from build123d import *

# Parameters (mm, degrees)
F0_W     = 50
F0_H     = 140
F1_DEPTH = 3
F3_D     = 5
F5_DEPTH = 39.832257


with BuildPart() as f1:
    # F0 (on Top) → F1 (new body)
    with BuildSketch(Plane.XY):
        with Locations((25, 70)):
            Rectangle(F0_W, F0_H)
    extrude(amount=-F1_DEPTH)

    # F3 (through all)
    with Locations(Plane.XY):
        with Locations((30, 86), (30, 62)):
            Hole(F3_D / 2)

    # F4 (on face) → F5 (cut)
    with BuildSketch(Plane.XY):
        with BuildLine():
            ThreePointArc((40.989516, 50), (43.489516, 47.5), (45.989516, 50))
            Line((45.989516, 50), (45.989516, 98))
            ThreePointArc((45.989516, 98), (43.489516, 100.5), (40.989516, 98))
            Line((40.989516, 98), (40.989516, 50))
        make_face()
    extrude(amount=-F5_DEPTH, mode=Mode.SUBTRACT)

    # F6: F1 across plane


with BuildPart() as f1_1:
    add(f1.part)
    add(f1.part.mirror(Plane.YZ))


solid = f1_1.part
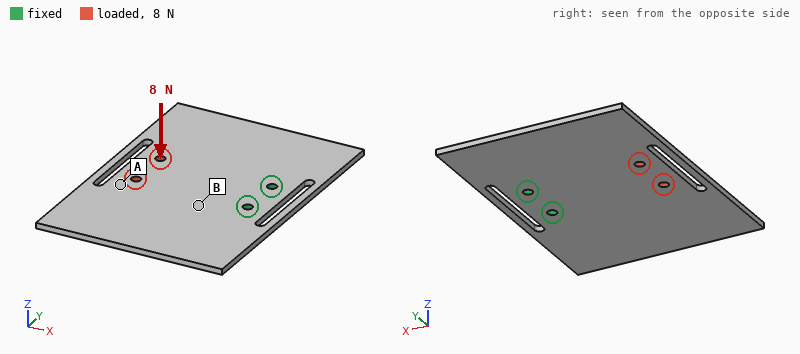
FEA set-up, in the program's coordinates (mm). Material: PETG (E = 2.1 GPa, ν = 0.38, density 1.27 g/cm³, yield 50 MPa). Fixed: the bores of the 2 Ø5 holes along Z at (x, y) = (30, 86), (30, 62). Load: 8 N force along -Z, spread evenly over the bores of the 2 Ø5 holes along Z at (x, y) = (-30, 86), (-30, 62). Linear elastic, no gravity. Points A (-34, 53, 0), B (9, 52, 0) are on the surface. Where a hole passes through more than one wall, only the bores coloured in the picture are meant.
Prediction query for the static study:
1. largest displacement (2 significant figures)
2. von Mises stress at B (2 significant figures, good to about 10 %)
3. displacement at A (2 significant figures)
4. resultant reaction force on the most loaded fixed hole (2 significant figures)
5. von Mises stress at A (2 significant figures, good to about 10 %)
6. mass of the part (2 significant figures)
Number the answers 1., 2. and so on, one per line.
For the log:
1. 1.9 mm
2. 1.7 MPa
3. 1.4 mm
4. 4.0 N
5. 0.50 MPa
6. 51 g
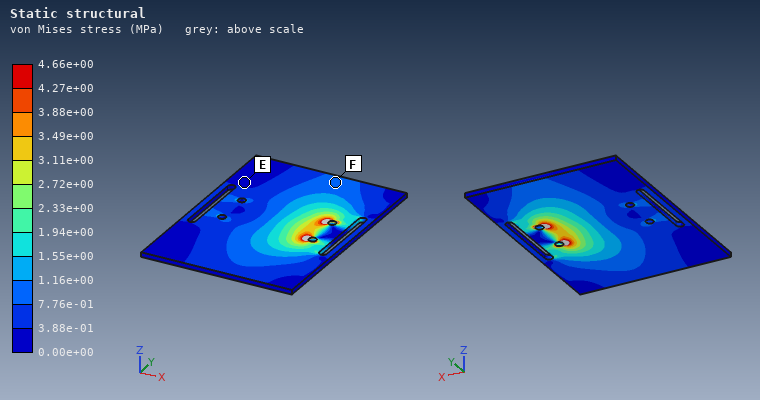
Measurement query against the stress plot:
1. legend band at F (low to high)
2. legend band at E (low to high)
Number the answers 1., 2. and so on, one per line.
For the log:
1. 7.76e-01 to 1.16e+00 MPa
2. 0.00e+00 to 3.88e-01 MPa
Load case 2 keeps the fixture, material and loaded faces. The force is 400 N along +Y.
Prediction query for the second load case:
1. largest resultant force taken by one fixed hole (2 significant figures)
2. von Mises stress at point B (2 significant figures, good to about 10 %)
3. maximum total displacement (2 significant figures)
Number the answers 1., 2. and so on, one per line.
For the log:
1. 880 N
2. 4.8 MPa
3. 1.4 mm
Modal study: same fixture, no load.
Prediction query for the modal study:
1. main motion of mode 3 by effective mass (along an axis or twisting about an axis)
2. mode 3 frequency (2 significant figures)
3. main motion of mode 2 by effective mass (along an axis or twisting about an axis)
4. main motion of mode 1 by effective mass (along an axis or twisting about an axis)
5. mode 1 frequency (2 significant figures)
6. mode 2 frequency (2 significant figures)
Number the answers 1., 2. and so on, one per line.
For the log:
1. along Z
2. 180 Hz
3. twisting about X
4. along Z
5. 81 Hz
6. 98 Hz
